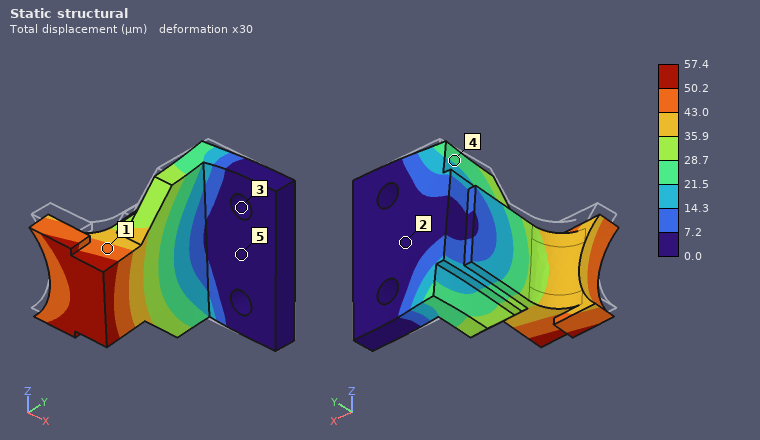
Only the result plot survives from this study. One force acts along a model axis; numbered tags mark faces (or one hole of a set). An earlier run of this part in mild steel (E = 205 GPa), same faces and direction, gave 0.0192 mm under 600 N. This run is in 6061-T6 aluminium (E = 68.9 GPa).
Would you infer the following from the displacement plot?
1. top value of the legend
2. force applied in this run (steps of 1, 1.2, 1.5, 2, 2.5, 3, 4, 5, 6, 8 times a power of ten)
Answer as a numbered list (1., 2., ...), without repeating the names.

1. 57.4 µm
2. 600 N
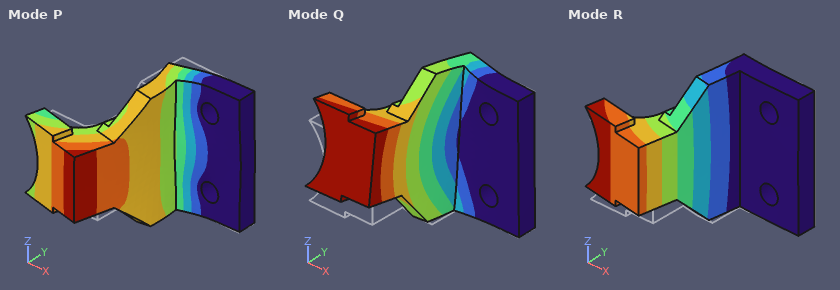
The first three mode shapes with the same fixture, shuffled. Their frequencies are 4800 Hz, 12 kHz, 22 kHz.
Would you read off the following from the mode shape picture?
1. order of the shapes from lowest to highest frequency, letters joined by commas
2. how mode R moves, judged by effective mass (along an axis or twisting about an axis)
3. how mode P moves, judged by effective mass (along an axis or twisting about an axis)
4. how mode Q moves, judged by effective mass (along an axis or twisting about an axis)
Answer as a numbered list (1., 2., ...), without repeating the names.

1. R, Q, P
2. along X
3. along Y
4. along Z
